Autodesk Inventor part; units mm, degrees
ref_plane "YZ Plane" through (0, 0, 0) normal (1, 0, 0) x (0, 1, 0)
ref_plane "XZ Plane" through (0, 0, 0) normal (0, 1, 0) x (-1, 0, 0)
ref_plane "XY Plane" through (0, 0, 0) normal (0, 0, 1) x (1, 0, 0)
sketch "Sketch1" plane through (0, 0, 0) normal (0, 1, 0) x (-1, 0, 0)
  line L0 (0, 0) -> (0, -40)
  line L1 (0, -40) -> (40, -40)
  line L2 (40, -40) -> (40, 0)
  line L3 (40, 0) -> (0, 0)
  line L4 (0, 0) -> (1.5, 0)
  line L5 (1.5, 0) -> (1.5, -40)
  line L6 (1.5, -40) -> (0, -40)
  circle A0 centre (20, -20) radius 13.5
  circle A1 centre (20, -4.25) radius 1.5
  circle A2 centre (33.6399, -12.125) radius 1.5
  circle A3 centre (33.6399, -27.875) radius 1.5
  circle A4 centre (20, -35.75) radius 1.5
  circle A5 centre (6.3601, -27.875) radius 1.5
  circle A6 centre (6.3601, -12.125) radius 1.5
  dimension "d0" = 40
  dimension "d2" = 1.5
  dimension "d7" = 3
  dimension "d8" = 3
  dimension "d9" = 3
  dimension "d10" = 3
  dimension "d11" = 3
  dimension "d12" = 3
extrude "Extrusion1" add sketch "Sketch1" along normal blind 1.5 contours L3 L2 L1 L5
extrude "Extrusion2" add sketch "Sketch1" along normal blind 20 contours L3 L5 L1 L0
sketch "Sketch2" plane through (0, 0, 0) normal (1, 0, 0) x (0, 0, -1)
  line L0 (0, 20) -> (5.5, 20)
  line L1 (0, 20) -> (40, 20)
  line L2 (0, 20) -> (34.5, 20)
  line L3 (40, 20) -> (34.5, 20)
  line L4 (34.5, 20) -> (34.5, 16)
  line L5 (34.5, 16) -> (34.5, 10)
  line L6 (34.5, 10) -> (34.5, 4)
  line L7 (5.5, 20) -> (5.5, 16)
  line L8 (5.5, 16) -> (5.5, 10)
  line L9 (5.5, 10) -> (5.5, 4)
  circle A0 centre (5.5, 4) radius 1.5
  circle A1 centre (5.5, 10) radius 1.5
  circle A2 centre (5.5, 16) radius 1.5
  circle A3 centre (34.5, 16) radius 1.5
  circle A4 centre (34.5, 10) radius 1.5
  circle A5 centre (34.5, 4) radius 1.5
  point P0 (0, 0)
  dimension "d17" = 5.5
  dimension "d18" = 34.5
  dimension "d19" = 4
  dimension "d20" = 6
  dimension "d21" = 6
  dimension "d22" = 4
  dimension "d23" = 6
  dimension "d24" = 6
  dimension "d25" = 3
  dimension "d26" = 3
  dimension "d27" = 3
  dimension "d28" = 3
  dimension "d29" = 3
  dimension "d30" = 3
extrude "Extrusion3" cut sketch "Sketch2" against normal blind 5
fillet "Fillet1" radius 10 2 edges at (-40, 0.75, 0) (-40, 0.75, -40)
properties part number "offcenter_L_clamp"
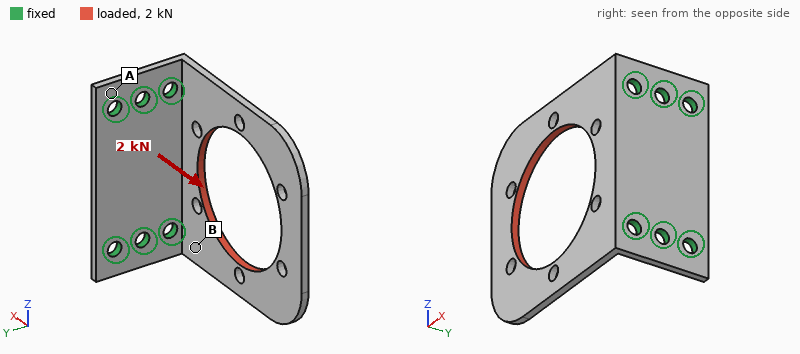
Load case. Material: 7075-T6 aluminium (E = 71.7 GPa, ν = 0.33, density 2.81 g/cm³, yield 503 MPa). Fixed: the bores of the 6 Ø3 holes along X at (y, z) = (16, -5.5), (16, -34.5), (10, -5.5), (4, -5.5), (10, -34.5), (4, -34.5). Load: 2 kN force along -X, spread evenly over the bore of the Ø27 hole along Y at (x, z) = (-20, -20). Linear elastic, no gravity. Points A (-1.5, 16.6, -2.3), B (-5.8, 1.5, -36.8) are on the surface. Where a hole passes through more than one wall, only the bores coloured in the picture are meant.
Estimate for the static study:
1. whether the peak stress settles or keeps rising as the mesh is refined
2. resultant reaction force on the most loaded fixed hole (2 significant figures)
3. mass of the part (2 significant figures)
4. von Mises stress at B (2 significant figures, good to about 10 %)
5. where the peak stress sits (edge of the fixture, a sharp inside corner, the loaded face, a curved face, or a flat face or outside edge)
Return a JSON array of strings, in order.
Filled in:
["keeps rising", "1.1 kN", "6.9 g", "80 MPa", "edge of the fixture"]
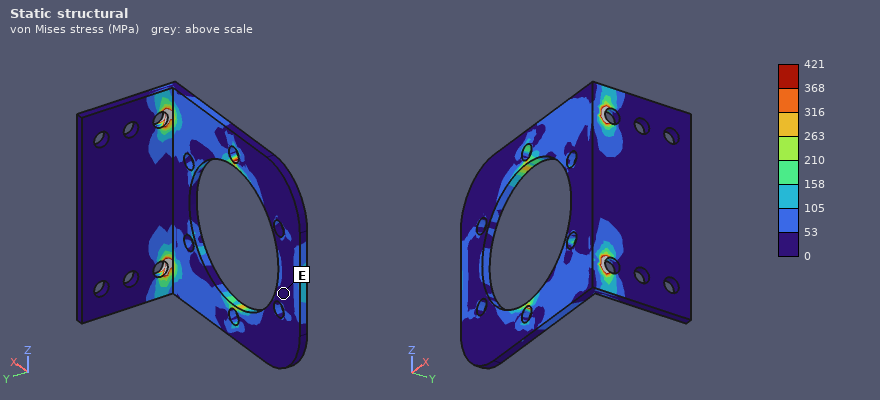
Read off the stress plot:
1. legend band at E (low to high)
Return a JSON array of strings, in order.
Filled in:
["0 to 53 MPa"]
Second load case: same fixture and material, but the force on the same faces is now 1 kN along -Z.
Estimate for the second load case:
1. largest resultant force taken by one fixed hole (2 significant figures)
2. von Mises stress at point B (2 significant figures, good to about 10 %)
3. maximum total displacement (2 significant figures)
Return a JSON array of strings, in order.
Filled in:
["720 N", "85 MPa", "0.27 mm"]
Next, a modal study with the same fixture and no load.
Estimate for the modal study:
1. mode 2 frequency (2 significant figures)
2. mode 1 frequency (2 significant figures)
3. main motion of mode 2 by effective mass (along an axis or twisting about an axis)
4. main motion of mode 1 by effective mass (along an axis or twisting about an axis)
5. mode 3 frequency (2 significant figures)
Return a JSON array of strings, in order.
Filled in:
["1600 Hz", "640 Hz", "twisting about X", "along Y", "3900 Hz"]
